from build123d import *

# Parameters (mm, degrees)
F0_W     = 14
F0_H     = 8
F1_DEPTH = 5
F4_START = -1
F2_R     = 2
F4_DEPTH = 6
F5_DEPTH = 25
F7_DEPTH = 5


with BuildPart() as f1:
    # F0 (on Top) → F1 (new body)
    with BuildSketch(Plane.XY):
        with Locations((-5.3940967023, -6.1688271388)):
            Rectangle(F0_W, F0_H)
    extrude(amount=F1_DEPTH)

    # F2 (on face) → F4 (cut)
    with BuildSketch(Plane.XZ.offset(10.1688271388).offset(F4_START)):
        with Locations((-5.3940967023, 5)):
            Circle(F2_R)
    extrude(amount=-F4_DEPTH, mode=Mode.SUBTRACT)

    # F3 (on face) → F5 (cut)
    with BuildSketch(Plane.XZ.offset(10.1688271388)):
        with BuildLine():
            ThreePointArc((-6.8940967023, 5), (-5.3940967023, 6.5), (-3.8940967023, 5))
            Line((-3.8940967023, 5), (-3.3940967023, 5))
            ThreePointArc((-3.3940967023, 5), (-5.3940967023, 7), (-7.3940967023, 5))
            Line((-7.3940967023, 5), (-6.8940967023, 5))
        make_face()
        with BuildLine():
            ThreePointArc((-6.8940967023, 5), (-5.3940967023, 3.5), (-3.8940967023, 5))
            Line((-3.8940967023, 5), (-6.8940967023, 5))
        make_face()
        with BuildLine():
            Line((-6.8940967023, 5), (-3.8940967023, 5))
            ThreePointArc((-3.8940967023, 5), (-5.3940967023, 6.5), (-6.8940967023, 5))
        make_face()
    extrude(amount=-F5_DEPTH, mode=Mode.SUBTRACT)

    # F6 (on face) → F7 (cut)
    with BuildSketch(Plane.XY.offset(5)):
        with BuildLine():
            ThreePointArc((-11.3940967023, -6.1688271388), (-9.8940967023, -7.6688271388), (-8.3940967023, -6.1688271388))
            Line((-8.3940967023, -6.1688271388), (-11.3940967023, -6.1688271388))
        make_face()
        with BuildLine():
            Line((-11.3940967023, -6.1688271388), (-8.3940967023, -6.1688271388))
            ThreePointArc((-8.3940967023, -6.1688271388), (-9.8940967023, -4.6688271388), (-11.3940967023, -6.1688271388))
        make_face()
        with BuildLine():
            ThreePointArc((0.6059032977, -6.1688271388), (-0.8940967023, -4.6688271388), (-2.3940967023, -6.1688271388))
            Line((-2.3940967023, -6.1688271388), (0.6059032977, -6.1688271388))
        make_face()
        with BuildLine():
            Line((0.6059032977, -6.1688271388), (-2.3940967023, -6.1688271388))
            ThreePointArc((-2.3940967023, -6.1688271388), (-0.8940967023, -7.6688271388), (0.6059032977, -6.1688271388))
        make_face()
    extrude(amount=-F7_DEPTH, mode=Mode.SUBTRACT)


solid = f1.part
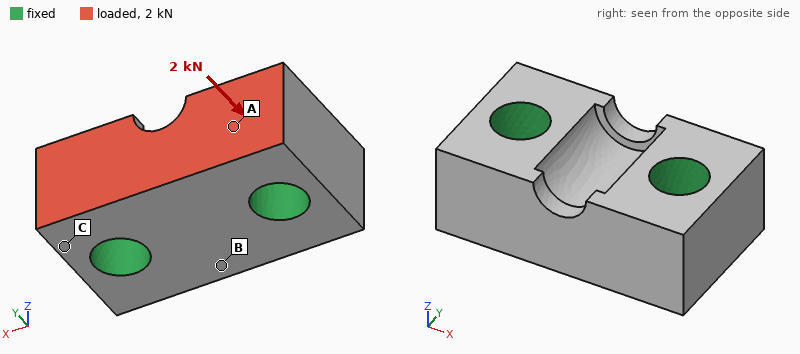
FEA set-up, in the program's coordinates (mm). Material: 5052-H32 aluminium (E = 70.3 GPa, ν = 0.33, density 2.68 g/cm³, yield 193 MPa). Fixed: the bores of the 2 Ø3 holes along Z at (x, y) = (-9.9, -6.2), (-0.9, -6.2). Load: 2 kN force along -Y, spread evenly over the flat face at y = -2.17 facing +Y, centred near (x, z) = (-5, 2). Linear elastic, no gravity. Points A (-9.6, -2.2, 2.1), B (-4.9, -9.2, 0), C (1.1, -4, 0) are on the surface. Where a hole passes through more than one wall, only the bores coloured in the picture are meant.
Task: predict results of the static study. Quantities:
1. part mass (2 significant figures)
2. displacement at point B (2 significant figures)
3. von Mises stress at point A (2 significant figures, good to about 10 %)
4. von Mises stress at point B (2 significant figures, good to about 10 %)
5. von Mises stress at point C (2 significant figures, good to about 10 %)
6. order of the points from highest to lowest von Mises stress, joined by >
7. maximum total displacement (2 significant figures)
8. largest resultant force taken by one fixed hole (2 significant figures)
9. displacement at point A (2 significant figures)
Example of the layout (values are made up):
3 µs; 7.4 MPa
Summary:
1.2 g; 0.91 µm; 39 MPa; 7.1 MPa; 23 MPa; A > C > B; 3.0 µm; 1.0 kN; 1.2 µm
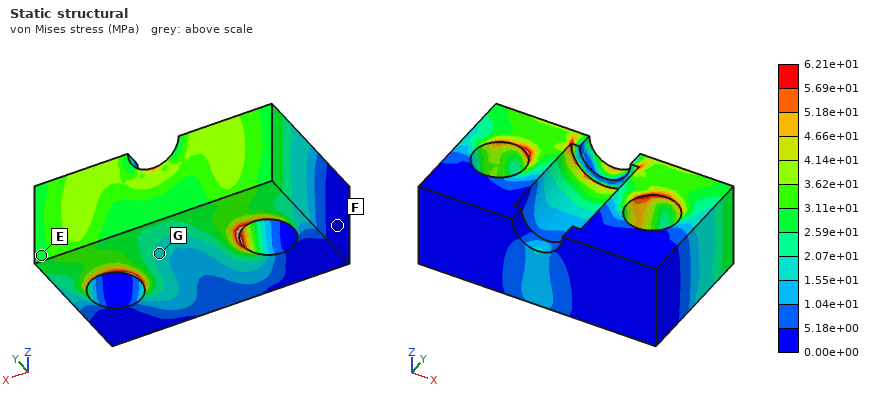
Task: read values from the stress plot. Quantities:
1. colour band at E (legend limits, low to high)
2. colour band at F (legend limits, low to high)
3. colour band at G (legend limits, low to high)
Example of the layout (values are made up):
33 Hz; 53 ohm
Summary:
2.59e+01 to 3.11e+01 MPa; 0.00e+00 to 5.18e+00 MPa; 1.55e+01 to 2.07e+01 MPa
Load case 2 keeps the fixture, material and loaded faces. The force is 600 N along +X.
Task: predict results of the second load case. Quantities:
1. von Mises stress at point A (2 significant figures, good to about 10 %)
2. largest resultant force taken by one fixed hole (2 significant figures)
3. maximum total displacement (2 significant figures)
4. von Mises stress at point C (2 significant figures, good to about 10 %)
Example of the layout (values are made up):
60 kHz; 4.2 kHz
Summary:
18 MPa; 330 N; 2.3 µm; 12 MPa
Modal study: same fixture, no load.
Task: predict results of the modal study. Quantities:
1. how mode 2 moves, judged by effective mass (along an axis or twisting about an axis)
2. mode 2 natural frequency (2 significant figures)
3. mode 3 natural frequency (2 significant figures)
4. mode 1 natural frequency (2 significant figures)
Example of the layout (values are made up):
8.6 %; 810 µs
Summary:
along Z; 170 kHz; 190 kHz; 160 kHz
